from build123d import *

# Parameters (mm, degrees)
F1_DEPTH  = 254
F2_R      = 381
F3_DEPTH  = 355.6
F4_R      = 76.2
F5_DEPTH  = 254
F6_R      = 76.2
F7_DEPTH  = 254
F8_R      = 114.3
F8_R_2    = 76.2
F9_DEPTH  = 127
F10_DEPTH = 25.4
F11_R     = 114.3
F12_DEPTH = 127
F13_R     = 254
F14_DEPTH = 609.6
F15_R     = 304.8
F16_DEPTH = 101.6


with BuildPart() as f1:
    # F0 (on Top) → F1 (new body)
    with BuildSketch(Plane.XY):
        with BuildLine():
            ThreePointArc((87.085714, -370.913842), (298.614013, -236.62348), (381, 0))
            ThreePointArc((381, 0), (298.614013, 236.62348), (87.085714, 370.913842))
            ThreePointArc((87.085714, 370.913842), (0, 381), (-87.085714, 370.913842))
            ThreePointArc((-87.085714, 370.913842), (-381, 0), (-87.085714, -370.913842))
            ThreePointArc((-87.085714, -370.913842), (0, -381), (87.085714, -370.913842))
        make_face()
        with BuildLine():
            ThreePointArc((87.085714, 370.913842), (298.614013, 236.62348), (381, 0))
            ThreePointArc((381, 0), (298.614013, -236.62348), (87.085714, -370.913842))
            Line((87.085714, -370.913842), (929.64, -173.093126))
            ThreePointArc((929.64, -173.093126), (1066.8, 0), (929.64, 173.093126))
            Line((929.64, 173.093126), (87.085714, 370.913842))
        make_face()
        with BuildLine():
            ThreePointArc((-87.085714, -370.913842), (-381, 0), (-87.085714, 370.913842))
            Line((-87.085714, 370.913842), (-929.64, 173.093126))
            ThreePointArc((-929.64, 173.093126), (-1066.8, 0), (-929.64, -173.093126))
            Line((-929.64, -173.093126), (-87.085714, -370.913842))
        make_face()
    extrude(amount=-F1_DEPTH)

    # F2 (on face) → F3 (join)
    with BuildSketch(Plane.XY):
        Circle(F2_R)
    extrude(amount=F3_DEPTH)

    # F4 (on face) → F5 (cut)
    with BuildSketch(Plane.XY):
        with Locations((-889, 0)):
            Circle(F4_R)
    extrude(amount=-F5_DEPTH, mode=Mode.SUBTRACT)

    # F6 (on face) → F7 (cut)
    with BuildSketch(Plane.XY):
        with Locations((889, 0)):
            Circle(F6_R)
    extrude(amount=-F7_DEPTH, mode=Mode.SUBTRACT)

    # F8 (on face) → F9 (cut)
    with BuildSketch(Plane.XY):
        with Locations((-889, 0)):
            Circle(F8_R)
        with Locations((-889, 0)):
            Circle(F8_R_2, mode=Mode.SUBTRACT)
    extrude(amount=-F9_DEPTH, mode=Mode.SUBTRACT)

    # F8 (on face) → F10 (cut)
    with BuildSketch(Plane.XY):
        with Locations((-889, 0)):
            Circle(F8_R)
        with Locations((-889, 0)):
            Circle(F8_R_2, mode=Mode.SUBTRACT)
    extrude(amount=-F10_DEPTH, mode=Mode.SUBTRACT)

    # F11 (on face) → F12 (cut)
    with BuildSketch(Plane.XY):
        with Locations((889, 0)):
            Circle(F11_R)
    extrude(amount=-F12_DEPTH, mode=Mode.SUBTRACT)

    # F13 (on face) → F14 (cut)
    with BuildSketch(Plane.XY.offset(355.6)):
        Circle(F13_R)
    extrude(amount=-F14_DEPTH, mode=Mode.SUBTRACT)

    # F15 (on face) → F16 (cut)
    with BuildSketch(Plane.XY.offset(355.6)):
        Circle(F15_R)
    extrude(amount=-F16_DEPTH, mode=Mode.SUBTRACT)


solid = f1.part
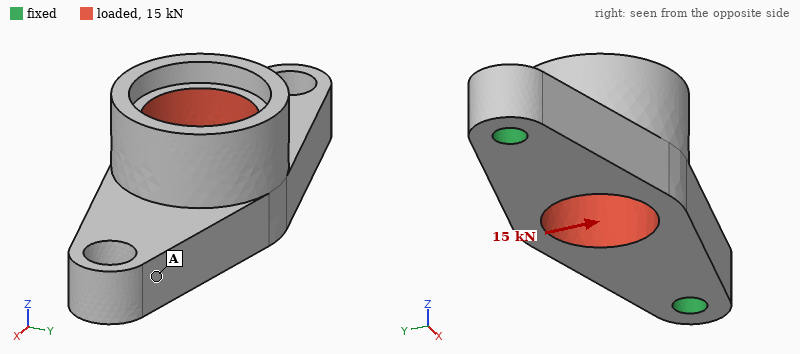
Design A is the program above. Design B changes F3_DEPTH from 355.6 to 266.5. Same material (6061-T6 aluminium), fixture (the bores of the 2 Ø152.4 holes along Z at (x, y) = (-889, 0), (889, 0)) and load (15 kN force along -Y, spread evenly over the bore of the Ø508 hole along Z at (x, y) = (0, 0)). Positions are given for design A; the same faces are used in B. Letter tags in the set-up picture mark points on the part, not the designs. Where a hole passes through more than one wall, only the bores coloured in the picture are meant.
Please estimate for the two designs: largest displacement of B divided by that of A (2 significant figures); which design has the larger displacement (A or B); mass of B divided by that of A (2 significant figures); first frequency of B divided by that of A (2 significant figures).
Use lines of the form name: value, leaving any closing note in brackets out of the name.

largest displacement of B divided by that of A: 0.90
which design has the larger displacement: A
mass of B divided by that of A: 0.95
first frequency of B divided by that of A: 1.1
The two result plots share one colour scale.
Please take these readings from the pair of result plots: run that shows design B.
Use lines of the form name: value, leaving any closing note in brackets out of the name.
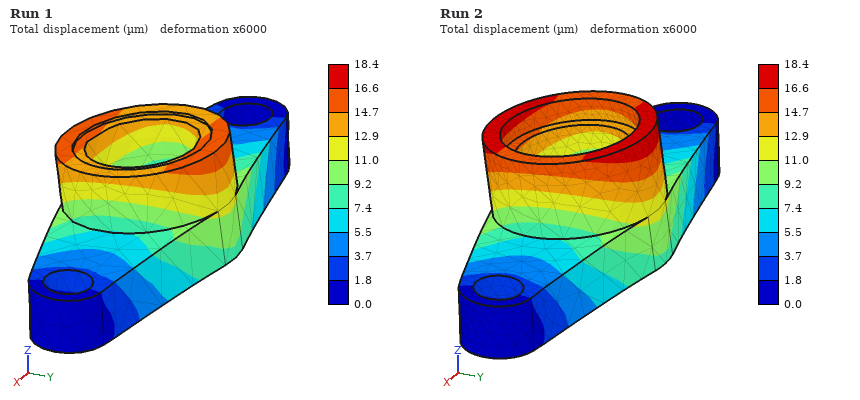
run that shows design B: Run 1
